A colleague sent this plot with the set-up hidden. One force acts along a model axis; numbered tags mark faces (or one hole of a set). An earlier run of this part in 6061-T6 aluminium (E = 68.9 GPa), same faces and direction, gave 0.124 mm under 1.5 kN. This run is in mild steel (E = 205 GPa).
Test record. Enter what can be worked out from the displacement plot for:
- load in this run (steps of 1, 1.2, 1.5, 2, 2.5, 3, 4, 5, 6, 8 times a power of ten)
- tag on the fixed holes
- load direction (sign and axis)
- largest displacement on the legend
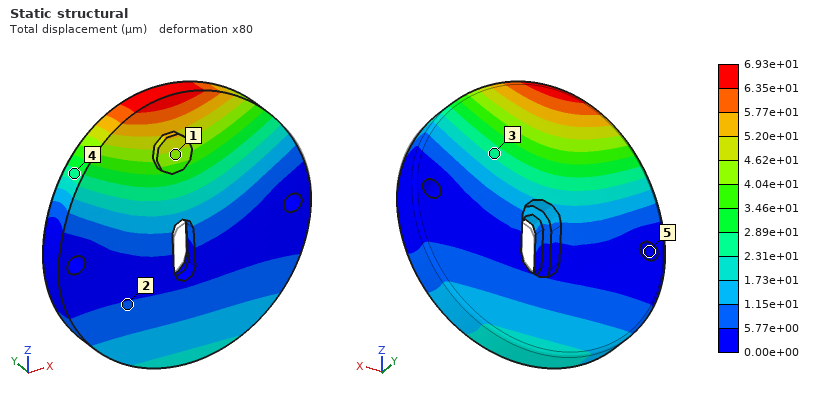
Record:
2.5 kN
5
+Y
6.93e+01 µm
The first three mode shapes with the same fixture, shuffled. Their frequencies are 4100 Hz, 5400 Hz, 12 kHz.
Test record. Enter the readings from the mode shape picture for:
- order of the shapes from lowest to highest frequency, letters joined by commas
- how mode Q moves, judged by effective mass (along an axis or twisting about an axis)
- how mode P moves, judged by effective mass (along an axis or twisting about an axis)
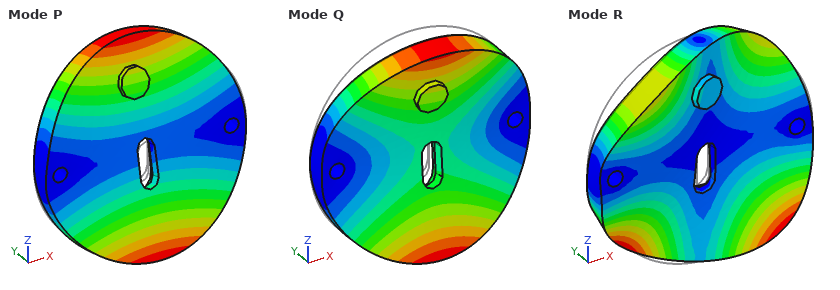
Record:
P, Q, R
along Y
twisting about X
